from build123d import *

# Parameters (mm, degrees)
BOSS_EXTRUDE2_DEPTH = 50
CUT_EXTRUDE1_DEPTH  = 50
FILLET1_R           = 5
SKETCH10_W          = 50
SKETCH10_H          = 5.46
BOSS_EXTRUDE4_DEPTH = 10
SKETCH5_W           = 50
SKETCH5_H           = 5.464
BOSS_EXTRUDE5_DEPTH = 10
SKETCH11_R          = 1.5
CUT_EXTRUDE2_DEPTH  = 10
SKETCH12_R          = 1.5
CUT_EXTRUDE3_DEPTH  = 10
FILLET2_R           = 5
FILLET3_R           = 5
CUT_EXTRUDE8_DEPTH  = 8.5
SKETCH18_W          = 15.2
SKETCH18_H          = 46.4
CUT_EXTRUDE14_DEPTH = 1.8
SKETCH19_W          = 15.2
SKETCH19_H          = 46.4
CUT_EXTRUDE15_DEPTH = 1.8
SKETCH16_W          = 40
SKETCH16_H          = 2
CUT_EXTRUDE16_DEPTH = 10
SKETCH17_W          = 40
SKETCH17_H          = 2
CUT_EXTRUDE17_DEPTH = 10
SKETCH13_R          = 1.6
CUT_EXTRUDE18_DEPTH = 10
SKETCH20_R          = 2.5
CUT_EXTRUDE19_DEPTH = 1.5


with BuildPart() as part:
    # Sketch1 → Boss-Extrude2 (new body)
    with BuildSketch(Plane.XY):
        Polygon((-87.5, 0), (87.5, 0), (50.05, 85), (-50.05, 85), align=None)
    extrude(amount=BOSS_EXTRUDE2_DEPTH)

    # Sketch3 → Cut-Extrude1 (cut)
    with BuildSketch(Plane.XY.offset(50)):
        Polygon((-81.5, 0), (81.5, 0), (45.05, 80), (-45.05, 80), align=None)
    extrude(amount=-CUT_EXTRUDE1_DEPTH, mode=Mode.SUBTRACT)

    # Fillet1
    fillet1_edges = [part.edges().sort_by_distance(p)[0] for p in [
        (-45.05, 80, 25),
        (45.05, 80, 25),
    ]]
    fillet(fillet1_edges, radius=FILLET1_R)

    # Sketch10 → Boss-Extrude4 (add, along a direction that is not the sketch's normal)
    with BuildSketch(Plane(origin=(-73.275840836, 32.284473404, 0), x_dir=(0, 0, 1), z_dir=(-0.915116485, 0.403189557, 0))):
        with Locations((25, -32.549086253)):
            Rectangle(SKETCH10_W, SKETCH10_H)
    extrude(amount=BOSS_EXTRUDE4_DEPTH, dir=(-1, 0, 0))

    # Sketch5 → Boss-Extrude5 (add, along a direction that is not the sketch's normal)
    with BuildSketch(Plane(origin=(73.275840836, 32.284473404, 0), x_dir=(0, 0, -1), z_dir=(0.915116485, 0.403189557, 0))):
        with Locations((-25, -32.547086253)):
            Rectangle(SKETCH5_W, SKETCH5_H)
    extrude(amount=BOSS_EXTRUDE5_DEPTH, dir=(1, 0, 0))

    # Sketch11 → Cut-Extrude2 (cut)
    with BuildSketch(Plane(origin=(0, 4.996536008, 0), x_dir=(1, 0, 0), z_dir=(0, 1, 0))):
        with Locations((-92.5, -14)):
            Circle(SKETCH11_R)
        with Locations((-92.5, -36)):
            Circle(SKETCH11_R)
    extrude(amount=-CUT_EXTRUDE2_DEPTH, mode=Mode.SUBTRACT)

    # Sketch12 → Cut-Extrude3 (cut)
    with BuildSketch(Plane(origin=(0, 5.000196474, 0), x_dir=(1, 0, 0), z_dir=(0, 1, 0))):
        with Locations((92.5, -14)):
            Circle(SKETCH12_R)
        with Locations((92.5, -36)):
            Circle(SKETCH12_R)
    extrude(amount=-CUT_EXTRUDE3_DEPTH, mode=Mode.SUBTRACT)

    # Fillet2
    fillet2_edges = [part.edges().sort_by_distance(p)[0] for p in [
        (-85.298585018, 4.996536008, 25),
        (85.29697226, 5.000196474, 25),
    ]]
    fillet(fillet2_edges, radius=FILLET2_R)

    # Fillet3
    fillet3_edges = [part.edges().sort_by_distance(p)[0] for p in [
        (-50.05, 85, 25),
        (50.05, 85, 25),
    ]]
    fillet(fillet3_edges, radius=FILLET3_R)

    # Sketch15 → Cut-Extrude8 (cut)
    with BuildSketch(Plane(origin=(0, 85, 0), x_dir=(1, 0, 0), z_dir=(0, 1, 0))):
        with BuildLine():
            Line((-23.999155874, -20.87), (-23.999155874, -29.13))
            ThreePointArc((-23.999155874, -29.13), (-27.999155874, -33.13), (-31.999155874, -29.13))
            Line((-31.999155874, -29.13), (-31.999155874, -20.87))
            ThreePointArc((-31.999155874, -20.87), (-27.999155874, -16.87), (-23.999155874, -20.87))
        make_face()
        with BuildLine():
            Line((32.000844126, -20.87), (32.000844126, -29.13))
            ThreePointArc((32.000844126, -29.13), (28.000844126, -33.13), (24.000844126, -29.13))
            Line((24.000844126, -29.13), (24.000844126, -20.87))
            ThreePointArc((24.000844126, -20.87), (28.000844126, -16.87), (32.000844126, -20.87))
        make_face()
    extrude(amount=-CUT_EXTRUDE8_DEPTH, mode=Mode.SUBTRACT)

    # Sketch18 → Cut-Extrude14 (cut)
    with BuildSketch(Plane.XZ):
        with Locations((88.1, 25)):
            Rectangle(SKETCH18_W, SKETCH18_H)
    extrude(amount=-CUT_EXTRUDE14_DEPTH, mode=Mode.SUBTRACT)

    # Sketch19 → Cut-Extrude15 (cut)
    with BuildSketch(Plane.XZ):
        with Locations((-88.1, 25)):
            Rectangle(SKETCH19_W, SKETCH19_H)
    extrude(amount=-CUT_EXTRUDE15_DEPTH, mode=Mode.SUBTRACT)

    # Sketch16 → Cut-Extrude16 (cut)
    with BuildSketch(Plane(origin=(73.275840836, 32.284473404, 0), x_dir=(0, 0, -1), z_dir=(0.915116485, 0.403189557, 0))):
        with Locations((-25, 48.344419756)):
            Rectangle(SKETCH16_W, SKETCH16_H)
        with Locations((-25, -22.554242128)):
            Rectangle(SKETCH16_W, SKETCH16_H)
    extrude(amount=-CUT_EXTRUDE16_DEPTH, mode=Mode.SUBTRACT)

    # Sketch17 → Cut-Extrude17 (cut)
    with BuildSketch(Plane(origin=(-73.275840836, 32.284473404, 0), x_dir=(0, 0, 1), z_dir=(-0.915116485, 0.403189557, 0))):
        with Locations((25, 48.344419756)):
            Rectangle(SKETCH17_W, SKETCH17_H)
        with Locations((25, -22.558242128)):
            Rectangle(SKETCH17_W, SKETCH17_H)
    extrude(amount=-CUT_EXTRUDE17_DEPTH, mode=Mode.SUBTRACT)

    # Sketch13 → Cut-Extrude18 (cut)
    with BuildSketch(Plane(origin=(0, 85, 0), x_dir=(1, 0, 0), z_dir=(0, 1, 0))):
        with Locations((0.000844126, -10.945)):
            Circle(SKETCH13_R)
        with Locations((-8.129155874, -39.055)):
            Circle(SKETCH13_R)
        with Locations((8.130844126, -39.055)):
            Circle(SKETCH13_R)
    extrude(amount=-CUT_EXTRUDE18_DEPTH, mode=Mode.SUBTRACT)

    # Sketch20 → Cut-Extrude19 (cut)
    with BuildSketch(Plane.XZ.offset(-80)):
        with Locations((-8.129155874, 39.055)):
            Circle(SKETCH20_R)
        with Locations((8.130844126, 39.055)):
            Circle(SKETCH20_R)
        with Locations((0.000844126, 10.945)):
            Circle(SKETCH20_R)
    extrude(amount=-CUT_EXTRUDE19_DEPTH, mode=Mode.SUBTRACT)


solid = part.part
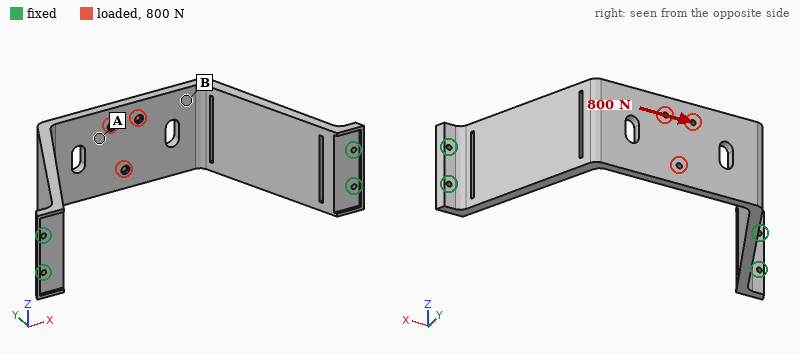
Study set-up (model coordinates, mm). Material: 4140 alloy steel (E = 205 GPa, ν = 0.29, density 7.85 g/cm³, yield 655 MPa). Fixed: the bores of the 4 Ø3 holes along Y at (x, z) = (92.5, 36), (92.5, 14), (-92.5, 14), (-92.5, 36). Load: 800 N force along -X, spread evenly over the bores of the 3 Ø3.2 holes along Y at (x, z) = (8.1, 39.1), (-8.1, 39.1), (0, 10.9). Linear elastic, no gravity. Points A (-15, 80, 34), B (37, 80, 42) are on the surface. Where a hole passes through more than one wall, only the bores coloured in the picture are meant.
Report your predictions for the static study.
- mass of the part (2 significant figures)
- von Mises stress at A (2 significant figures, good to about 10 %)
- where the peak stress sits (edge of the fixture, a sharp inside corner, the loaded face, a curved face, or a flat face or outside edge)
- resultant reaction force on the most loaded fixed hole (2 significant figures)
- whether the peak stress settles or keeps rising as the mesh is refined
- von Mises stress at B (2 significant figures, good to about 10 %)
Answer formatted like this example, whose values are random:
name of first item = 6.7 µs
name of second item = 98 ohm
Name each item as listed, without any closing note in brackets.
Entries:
mass of the part = 610 g
von Mises stress at A = 21 MPa
where the peak stress sits = a sharp inside corner
resultant reaction force on the most loaded fixed hole = 300 N
whether the peak stress settles or keeps rising as the mesh is refined = keeps rising
von Mises stress at B = 65 MPa
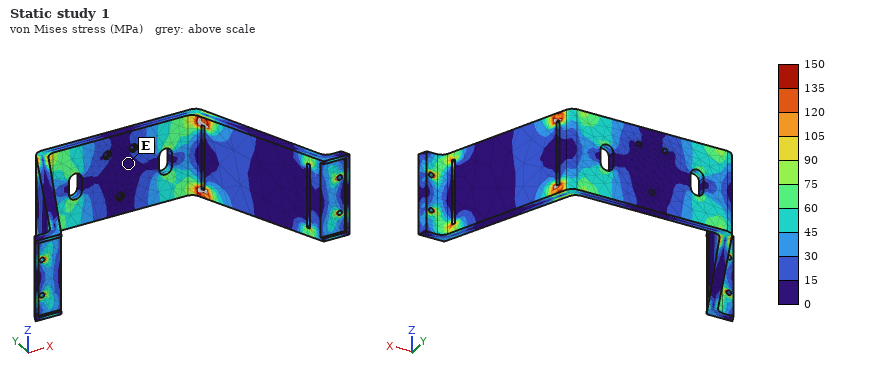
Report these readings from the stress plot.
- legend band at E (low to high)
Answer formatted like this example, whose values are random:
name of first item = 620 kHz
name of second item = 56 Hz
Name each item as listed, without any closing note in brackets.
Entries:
legend band at E = 0 to 15 MPa
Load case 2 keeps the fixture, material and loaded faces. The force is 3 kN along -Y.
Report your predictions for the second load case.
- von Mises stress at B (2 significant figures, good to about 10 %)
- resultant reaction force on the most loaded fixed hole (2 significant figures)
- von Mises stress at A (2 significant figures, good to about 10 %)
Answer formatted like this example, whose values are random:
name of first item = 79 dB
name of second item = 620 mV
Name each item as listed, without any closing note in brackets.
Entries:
von Mises stress at B = 67 MPa
resultant reaction force on the most loaded fixed hole = 1.3 kN
von Mises stress at A = 130 MPa
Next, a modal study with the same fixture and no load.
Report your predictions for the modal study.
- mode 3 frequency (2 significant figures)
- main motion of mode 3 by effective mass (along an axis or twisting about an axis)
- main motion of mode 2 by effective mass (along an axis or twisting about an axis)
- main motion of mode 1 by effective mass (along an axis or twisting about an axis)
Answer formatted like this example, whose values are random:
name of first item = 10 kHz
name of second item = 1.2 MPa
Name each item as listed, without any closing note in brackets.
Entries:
mode 3 frequency = 1000 Hz
main motion of mode 3 by effective mass = twisting about Y
main motion of mode 2 by effective mass = along Z
main motion of mode 1 by effective mass = along X
